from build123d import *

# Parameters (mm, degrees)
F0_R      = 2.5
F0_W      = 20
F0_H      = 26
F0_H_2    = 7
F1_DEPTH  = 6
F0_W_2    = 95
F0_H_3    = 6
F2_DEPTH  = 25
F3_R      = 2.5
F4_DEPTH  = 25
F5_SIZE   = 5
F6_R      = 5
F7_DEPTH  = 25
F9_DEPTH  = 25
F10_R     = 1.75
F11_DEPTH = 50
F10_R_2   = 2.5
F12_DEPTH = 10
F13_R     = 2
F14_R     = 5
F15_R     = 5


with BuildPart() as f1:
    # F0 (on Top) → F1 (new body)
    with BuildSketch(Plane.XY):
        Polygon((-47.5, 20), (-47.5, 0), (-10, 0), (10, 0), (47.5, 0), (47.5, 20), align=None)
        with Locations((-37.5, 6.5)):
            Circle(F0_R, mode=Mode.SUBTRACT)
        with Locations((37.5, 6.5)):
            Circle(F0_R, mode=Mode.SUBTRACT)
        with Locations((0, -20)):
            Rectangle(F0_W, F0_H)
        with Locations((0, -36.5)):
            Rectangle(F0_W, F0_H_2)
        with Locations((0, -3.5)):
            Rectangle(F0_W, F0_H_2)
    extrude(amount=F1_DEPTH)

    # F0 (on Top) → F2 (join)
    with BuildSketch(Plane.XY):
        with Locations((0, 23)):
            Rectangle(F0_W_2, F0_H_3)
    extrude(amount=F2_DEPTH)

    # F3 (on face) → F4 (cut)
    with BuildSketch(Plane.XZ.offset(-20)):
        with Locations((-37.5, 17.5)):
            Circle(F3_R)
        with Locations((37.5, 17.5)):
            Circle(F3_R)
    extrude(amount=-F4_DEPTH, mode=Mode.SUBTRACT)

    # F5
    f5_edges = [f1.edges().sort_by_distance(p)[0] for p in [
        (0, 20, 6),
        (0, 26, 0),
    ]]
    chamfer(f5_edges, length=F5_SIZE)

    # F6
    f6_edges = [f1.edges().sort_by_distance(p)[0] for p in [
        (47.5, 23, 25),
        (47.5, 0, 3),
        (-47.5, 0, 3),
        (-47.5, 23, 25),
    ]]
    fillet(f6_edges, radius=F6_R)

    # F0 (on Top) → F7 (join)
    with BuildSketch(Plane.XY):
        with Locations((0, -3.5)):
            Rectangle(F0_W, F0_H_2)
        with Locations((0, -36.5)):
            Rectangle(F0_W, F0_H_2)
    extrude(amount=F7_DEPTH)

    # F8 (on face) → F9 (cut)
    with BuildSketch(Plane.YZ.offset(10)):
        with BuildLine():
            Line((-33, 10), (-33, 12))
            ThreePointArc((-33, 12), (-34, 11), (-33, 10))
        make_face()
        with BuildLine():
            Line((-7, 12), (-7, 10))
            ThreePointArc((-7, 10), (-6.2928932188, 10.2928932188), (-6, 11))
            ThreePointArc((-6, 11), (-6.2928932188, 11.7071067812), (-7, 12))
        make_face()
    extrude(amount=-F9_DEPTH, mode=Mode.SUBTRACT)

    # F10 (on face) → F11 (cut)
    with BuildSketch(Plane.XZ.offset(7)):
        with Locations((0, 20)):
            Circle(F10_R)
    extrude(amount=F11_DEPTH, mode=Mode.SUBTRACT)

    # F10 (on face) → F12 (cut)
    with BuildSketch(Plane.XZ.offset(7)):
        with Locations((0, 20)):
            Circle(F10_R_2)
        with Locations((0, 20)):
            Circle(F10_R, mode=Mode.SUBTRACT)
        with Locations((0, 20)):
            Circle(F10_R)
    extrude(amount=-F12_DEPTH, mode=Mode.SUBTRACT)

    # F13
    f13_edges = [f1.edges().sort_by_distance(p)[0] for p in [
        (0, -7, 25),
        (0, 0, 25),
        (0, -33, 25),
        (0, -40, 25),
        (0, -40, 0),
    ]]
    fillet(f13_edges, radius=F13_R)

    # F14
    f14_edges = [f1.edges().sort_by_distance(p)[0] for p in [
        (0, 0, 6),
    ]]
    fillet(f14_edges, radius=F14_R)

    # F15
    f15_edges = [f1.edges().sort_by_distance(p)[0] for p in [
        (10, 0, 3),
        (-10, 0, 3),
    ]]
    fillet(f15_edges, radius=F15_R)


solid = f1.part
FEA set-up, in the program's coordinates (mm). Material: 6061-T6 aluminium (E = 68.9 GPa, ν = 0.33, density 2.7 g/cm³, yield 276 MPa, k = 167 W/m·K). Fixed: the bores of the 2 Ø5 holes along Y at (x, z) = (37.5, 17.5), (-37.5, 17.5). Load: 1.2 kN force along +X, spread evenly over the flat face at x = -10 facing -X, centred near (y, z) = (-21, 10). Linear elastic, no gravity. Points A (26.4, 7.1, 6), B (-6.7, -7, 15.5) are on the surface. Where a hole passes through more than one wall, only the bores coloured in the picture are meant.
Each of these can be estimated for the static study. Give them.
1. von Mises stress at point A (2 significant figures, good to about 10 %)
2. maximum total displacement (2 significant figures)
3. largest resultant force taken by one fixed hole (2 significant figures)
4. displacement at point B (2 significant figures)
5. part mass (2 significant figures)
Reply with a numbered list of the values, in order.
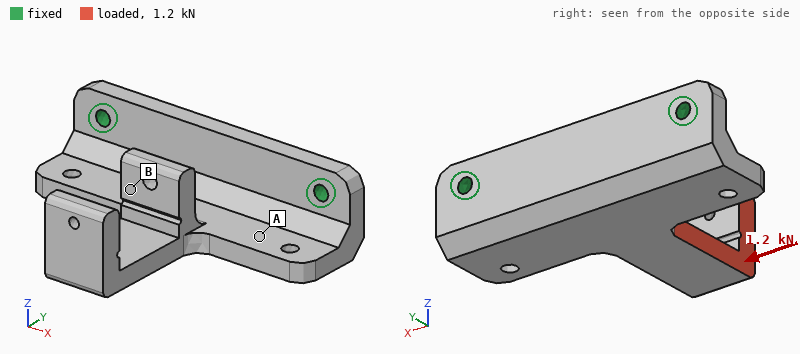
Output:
1. 18 MPa
2. 0.24 mm
3. 920 N
4. 0.055 mm
5. 94 g
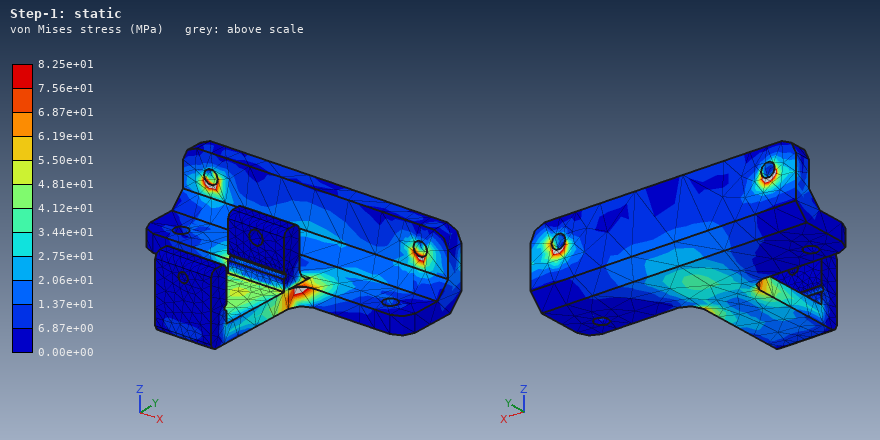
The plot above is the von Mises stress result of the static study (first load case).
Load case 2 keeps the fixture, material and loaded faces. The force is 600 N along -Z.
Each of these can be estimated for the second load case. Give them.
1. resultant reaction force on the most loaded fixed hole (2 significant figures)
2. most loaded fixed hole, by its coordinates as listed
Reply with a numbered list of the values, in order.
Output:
1. 460 N
2. (-37.5, 17.5)
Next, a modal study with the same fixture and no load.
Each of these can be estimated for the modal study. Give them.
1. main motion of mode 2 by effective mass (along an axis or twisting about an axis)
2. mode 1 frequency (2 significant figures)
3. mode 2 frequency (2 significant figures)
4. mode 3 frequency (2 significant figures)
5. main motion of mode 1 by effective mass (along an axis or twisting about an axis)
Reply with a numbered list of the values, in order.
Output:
1. along X
2. 990 Hz
3. 2800 Hz
4. 3100 Hz
5. along Z
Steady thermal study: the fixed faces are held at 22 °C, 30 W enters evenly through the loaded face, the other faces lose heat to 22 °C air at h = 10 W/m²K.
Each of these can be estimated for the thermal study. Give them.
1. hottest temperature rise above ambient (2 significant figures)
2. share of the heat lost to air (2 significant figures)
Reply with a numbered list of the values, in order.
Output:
1. 56 K
2. 7.9 %
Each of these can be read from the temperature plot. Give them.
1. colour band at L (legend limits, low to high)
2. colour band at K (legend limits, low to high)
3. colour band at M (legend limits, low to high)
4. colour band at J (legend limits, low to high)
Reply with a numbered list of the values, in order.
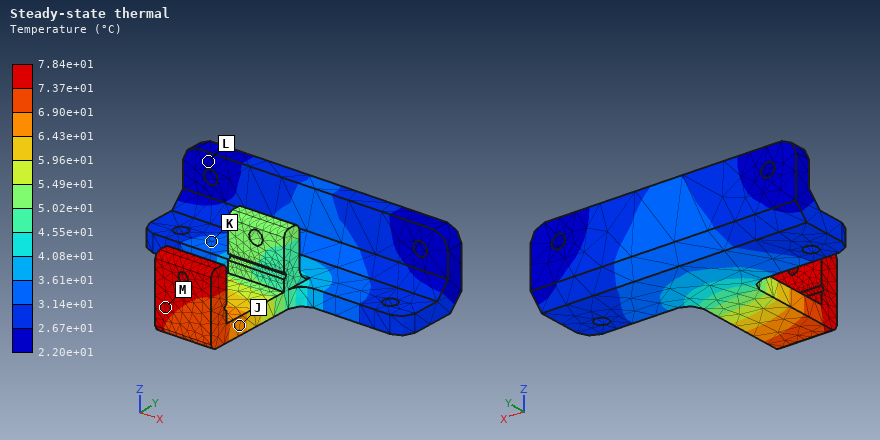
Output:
1. 2.20e+01 to 2.67e+01 °C
2. 3.14e+01 to 3.61e+01 °C
3. 7.37e+01 to 7.84e+01 °C
4. 6.43e+01 to 6.90e+01 °C
